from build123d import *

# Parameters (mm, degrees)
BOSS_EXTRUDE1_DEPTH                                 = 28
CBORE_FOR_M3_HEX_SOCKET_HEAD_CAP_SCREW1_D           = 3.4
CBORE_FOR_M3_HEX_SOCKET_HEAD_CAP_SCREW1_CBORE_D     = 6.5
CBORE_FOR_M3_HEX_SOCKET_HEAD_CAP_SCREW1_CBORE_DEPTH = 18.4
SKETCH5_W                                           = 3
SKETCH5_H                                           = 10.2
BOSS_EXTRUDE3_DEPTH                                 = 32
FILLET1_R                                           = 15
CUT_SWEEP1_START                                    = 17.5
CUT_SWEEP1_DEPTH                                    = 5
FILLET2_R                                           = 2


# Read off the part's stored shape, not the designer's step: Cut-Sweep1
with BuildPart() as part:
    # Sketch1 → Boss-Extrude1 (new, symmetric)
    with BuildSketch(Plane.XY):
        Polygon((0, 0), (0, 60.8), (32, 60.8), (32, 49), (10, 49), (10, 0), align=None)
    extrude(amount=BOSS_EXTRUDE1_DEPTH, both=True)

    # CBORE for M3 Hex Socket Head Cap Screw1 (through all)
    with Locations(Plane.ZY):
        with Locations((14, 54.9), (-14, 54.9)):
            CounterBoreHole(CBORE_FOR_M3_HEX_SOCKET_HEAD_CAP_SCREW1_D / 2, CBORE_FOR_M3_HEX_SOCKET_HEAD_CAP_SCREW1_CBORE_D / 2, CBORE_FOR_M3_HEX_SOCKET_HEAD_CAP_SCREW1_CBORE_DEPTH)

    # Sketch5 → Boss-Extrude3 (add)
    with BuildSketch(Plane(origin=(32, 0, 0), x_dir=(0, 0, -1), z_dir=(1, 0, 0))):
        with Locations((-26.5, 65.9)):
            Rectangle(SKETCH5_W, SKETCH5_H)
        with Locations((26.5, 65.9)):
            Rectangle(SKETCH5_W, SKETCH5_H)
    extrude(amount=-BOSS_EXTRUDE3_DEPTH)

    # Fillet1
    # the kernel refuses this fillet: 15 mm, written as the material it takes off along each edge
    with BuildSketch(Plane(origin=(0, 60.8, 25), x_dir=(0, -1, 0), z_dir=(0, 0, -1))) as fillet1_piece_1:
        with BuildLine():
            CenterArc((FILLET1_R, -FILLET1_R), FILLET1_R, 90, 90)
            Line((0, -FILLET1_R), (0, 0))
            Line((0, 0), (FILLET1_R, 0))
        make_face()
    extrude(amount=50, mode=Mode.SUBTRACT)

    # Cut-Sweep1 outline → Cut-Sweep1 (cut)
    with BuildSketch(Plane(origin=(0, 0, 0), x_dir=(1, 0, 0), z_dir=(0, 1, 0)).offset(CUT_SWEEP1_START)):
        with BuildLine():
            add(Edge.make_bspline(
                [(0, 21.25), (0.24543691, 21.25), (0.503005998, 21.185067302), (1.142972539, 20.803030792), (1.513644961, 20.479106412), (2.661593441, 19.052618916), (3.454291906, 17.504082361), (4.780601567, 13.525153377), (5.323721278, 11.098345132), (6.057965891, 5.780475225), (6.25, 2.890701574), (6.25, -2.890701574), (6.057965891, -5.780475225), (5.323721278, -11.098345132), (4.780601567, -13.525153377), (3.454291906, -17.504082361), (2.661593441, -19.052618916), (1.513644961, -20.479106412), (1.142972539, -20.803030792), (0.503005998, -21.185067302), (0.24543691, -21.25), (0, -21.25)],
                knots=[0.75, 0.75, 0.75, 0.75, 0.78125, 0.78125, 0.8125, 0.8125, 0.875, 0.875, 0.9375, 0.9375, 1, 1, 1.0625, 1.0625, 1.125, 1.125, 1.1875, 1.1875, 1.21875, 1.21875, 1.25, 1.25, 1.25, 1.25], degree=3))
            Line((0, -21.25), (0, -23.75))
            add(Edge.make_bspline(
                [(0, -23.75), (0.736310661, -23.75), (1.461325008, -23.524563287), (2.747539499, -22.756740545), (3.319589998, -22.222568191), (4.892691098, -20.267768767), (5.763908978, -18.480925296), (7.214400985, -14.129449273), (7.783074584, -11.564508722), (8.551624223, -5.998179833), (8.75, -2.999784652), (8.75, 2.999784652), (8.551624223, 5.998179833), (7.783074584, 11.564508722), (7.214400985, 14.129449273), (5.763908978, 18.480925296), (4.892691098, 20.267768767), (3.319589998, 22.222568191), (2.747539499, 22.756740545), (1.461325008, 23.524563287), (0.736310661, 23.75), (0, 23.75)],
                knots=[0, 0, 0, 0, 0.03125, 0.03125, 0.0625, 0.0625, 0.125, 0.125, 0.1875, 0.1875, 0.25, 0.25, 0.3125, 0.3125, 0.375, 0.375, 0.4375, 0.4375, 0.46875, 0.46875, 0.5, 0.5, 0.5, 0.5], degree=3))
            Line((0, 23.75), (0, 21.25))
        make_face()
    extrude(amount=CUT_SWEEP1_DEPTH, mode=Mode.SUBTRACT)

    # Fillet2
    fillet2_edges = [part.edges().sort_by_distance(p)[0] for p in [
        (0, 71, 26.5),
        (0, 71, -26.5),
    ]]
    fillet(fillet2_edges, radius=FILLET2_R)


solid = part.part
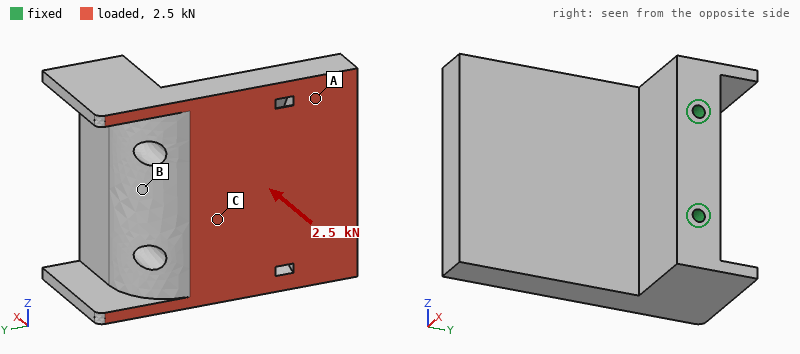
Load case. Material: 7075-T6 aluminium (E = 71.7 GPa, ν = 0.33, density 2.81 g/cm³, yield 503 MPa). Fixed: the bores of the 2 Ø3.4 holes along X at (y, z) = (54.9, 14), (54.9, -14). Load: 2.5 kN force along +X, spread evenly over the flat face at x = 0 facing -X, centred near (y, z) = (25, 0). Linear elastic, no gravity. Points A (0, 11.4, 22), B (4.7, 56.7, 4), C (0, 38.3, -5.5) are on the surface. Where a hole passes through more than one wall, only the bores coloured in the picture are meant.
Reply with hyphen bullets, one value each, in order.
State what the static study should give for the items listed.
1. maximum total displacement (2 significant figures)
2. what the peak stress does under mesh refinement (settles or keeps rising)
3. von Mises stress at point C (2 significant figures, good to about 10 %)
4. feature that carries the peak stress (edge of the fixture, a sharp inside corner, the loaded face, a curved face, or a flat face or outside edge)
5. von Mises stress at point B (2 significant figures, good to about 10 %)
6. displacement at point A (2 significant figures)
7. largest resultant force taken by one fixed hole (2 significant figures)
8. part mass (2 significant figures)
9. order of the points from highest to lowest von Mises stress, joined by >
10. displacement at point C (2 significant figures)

- 0.36 mm
- keeps rising
- 37 MPa
- edge of the fixture
- 51 MPa
- 0.28 mm
- 1.3 kN
- 130 g
- B > C > A
- 0.11 mm
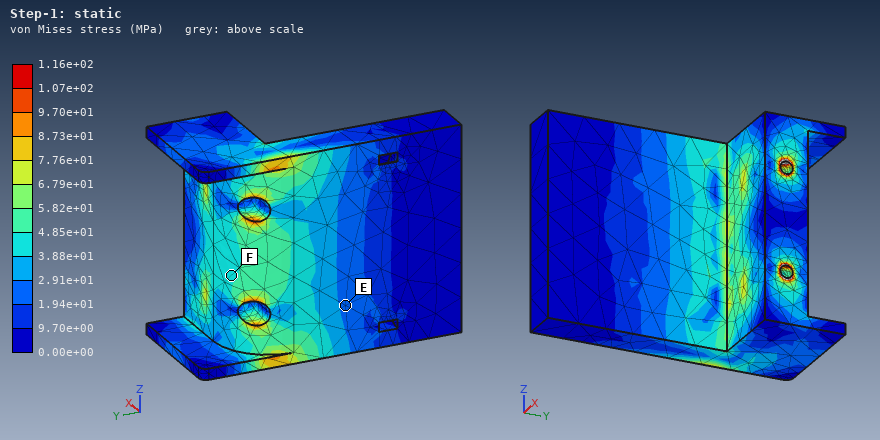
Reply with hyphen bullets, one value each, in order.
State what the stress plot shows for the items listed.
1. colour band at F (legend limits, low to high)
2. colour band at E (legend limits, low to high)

- 3.88e+01 to 4.85e+01 MPa
- 1.94e+01 to 2.91e+01 MPa
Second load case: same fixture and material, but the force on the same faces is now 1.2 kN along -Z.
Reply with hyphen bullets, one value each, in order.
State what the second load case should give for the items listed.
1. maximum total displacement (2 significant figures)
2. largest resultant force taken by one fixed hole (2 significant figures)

- 39 µm
- 1.5 kN
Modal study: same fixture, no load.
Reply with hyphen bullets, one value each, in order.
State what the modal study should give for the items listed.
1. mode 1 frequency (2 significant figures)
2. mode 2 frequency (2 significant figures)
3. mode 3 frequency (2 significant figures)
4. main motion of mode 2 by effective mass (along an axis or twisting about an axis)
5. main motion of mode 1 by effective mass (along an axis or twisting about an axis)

- 1800 Hz
- 3400 Hz
- 5600 Hz
- along Z
- along X
